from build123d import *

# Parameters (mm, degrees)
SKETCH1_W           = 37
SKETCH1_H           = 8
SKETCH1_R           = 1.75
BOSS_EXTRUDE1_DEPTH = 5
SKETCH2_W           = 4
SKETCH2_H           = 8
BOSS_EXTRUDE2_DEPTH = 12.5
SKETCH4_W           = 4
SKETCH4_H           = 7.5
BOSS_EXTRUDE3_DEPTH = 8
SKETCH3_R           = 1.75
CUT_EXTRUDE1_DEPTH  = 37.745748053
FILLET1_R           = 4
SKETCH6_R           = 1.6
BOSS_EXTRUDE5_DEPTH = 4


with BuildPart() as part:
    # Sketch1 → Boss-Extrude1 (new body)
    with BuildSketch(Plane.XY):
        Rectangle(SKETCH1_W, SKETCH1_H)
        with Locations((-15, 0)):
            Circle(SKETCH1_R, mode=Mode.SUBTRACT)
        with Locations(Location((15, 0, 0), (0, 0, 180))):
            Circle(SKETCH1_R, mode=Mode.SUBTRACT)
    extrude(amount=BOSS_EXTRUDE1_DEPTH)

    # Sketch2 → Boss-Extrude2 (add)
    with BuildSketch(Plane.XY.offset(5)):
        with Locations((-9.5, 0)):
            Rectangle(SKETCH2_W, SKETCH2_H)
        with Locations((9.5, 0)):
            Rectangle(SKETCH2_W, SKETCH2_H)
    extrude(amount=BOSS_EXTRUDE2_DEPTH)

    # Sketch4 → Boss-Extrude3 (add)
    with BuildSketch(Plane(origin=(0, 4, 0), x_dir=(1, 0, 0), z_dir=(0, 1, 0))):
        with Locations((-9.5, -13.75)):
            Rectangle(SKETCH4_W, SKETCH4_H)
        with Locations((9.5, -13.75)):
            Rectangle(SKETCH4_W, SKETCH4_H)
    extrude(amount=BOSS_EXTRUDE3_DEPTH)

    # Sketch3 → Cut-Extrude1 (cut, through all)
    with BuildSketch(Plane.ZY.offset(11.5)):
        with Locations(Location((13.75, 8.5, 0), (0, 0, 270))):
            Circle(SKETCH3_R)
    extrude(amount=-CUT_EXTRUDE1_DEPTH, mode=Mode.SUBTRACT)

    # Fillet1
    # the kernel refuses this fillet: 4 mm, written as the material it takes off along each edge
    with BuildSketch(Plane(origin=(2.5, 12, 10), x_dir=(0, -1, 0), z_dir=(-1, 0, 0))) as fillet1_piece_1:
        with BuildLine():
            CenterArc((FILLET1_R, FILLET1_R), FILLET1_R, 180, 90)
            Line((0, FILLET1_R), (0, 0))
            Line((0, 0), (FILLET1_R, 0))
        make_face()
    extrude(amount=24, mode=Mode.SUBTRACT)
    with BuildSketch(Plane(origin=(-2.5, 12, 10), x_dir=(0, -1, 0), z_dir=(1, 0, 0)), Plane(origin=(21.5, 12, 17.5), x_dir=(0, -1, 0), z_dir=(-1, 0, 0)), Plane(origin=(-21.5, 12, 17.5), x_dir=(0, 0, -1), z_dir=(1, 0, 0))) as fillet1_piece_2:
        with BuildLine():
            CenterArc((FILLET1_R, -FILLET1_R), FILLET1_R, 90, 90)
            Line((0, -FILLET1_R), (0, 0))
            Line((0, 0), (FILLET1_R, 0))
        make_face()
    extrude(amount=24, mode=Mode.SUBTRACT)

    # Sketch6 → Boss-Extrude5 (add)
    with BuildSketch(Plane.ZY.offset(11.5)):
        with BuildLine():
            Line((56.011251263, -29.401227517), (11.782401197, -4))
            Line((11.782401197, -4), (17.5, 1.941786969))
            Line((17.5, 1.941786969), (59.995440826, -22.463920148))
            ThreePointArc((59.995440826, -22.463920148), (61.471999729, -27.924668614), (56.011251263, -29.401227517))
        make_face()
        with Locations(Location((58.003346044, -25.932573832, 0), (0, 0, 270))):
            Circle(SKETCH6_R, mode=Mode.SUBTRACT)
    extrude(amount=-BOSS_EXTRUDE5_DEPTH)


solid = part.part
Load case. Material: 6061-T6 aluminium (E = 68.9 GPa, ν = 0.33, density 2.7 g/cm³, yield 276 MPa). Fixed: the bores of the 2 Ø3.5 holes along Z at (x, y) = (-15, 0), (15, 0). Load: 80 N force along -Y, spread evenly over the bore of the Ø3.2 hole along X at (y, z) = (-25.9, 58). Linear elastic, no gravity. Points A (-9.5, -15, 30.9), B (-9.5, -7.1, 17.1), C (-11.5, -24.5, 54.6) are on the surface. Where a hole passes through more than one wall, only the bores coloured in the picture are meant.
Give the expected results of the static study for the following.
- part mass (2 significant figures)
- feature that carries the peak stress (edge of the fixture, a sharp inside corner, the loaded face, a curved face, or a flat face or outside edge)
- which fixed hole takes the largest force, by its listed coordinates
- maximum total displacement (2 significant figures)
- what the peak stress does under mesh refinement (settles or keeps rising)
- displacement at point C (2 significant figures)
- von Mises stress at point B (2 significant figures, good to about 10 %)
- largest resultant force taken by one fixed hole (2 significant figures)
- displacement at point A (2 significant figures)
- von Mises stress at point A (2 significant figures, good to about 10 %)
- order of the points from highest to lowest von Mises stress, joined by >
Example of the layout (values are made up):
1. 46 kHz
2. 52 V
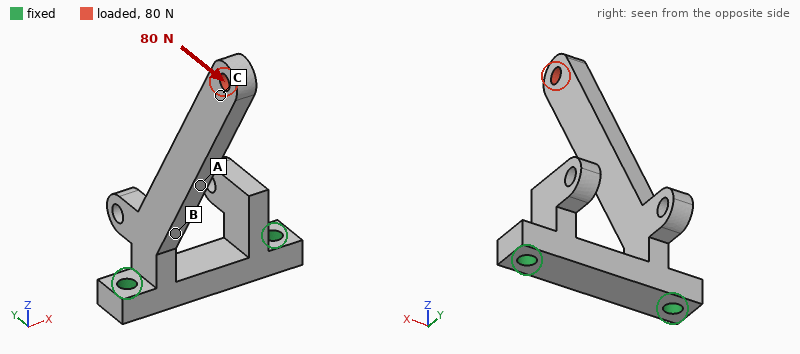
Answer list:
1. 11 g
2. edge of the fixture
3. (-15, 0)
4. 0.64 mm
5. keeps rising
6. 0.53 mm
7. 71 MPa
8. 86 N
9. 0.23 mm
10. 46 MPa
11. B > A > C
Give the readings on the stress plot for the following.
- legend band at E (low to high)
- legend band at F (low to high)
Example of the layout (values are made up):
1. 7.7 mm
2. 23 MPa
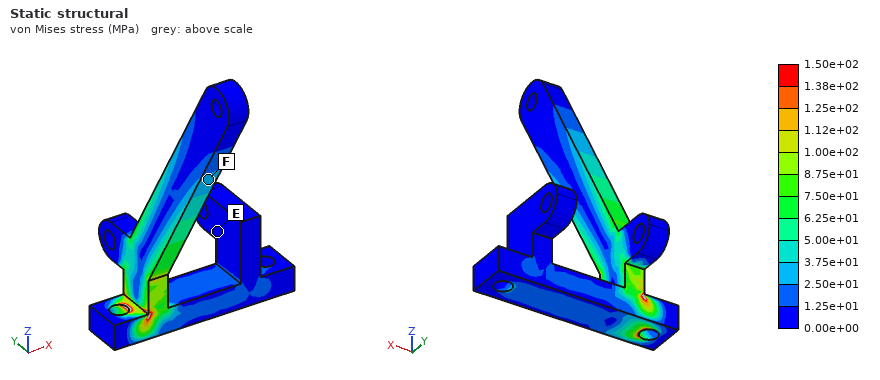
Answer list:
1. 0.00e+00 to 1.25e+01 MPa
2. 2.50e+01 to 3.75e+01 MPa
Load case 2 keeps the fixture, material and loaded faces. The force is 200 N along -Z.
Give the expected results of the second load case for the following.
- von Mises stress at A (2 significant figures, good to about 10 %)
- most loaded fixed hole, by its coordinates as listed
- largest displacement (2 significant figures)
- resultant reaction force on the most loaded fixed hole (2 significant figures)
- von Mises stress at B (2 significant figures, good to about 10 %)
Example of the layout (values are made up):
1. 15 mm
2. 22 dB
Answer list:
1. 73 MPa
2. (-15, 0)
3. 0.84 mm
4. 180 N
5. 110 MPa
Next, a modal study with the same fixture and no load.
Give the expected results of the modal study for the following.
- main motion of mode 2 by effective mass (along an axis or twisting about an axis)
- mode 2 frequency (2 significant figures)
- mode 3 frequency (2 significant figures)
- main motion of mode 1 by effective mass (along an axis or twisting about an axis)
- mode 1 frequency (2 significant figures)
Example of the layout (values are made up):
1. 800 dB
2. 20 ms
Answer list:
1. along Y
2. 1400 Hz
3. 4800 Hz
4. along X
5. 810 Hz
